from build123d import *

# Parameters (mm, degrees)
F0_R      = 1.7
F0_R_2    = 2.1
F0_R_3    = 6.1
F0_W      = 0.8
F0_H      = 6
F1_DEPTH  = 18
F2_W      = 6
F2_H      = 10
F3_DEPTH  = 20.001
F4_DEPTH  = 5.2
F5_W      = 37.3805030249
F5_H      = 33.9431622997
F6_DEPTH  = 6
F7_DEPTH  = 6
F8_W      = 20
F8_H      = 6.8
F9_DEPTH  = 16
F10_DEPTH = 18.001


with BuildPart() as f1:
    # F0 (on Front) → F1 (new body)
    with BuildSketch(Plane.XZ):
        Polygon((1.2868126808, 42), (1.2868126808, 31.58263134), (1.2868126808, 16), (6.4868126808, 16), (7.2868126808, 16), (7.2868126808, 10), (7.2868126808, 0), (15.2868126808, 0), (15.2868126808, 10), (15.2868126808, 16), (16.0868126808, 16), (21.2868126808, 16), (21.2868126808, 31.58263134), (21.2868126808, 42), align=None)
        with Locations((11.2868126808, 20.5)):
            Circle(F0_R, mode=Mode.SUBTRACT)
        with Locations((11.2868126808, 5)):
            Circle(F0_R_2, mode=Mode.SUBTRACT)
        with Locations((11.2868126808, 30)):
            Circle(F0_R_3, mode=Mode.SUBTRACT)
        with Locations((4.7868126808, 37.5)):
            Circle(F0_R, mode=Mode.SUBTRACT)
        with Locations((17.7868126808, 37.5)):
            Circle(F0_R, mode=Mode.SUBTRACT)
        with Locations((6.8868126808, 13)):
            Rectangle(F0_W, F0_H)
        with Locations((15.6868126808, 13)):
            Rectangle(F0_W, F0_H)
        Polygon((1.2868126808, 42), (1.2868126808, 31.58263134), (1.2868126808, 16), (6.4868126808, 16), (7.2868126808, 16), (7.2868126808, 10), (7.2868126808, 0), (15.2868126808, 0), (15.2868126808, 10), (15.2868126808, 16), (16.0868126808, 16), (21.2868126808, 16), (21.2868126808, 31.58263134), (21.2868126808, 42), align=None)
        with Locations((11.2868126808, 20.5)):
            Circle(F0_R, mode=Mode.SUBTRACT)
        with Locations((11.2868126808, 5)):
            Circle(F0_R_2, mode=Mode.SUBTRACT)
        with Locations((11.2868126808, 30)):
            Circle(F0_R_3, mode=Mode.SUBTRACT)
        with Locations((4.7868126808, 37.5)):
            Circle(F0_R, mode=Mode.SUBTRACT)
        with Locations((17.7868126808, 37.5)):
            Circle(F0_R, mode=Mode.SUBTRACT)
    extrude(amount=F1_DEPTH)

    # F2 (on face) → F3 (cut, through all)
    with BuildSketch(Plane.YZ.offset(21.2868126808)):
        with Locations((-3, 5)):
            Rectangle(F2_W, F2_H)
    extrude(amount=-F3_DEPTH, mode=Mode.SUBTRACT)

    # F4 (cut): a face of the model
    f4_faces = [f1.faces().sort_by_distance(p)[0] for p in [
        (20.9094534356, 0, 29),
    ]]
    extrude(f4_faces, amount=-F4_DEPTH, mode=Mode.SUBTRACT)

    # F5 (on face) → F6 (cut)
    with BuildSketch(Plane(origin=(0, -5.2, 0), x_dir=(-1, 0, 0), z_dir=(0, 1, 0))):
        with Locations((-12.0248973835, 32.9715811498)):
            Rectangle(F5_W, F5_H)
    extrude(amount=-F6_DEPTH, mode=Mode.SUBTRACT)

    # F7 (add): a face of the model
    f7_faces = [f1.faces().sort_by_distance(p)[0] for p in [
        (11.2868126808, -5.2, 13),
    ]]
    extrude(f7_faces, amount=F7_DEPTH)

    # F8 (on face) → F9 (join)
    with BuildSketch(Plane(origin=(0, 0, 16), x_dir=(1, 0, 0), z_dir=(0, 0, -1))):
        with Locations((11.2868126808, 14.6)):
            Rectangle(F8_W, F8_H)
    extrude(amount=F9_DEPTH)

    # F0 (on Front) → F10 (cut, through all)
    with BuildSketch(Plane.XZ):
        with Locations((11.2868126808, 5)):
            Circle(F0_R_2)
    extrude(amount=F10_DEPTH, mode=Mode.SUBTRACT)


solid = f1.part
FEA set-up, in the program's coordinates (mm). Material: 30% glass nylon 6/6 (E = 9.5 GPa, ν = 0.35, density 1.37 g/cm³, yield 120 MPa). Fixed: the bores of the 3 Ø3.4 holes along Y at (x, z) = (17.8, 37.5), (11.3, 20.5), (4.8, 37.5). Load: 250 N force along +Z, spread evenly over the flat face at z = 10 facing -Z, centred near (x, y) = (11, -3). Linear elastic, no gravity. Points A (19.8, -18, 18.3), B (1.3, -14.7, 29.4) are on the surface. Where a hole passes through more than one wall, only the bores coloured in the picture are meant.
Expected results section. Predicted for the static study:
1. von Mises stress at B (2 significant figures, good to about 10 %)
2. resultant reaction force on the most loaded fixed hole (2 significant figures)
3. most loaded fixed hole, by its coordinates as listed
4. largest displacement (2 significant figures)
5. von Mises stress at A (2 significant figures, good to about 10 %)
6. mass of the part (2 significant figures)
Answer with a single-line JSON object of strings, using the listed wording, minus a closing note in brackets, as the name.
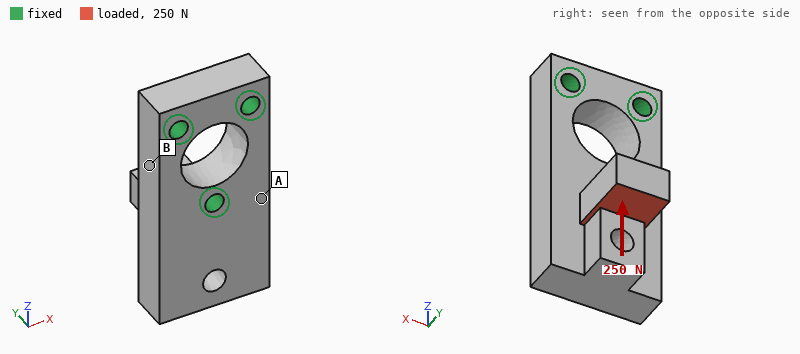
{"von Mises stress at B": "3.2 MPa", "resultant reaction force on the most loaded fixed hole": "220 N", "most loaded fixed hole, by its coordinates as listed": "(11.3, 20.5)", "largest displacement": "0.12 mm", "von Mises stress at A": "11 MPa", "mass of the part": "7.8 g"}
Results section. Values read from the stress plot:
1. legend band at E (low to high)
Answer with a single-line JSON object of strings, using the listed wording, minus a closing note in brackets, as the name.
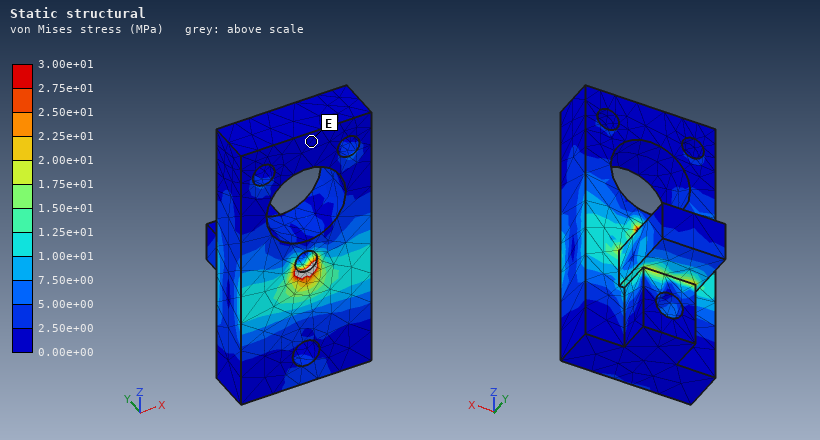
{"legend band at E": "0.00e+00 to 2.50e+00 MPa"}
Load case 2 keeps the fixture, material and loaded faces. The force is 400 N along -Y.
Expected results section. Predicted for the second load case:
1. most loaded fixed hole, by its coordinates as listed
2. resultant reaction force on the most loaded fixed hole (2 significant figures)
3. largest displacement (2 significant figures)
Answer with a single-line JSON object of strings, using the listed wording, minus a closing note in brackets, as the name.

{"most loaded fixed hole, by its coordinates as listed": "(11.3, 20.5)", "resultant reaction force on the most loaded fixed hole": "470 N", "largest displacement": "0.13 mm"}
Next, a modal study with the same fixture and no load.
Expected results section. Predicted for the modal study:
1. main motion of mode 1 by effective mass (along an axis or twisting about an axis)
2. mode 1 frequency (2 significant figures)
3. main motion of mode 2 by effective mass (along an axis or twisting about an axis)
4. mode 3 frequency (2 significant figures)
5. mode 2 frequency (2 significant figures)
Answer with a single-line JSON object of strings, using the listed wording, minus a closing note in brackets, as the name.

{"main motion of mode 1 by effective mass": "along Y", "mode 1 frequency": "4900 Hz", "main motion of mode 2 by effective mass": "along X", "mode 3 frequency": "8900 Hz", "mode 2 frequency": "7200 Hz"}
